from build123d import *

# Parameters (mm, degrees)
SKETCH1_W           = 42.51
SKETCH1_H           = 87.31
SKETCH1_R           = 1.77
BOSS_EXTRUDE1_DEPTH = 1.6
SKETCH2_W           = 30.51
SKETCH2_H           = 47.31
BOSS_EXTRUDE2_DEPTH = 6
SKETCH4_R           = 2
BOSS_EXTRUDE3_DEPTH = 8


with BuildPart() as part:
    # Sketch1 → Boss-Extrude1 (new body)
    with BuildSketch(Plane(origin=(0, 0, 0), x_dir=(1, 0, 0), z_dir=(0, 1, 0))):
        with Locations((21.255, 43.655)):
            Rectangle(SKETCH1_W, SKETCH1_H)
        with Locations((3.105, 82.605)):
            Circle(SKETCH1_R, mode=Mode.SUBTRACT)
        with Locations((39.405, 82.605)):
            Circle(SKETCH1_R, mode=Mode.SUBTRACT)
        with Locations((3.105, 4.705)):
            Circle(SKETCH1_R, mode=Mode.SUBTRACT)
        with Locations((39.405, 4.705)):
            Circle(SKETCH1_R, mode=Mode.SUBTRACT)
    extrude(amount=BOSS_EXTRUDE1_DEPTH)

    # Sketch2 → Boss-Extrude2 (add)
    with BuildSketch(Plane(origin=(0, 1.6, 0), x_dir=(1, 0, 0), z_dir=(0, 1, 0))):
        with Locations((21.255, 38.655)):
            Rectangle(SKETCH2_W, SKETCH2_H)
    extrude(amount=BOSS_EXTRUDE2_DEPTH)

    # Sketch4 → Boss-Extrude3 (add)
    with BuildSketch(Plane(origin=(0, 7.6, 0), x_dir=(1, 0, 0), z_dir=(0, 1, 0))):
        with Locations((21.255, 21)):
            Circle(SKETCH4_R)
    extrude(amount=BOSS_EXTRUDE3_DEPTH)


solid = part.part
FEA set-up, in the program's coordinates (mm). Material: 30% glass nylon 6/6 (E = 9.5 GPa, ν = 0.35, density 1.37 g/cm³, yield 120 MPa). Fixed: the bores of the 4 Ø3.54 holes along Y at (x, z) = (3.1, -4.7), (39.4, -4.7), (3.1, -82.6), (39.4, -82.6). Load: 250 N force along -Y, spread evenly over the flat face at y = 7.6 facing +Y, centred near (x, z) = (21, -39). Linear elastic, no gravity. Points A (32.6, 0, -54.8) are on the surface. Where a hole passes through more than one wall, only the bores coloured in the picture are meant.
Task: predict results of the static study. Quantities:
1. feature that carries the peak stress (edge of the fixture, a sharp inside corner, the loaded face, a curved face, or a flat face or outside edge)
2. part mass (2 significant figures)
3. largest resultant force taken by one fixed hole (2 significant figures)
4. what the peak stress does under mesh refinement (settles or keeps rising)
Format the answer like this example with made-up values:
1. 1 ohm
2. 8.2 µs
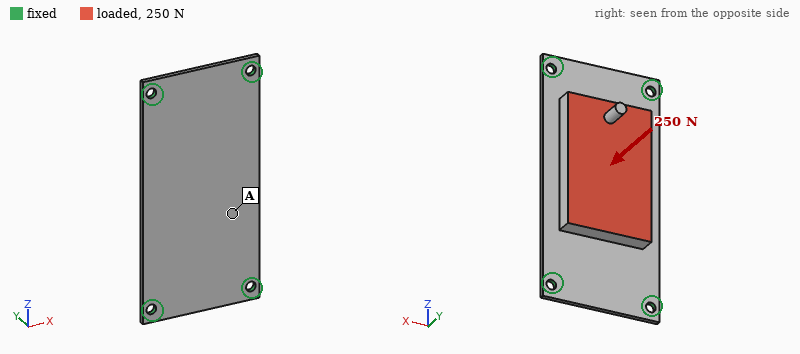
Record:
1. edge of the fixture
2. 20 g
3. 110 N
4. keeps rising
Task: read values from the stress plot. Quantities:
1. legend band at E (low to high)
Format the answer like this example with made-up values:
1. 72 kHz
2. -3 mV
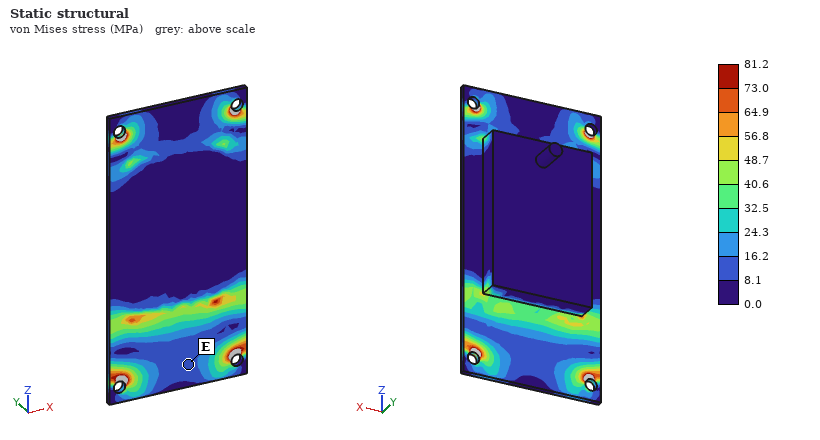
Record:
1. 8.1 to 16.2 MPa
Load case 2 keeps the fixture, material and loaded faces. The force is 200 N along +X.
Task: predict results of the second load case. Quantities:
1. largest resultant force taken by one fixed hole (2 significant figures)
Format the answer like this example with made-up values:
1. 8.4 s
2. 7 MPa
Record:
1. 98 N
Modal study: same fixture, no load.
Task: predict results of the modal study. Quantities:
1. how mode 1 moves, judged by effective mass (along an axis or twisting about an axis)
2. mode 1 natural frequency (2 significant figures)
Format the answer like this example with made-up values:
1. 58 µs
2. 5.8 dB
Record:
1. along Y
2. 790 Hz
